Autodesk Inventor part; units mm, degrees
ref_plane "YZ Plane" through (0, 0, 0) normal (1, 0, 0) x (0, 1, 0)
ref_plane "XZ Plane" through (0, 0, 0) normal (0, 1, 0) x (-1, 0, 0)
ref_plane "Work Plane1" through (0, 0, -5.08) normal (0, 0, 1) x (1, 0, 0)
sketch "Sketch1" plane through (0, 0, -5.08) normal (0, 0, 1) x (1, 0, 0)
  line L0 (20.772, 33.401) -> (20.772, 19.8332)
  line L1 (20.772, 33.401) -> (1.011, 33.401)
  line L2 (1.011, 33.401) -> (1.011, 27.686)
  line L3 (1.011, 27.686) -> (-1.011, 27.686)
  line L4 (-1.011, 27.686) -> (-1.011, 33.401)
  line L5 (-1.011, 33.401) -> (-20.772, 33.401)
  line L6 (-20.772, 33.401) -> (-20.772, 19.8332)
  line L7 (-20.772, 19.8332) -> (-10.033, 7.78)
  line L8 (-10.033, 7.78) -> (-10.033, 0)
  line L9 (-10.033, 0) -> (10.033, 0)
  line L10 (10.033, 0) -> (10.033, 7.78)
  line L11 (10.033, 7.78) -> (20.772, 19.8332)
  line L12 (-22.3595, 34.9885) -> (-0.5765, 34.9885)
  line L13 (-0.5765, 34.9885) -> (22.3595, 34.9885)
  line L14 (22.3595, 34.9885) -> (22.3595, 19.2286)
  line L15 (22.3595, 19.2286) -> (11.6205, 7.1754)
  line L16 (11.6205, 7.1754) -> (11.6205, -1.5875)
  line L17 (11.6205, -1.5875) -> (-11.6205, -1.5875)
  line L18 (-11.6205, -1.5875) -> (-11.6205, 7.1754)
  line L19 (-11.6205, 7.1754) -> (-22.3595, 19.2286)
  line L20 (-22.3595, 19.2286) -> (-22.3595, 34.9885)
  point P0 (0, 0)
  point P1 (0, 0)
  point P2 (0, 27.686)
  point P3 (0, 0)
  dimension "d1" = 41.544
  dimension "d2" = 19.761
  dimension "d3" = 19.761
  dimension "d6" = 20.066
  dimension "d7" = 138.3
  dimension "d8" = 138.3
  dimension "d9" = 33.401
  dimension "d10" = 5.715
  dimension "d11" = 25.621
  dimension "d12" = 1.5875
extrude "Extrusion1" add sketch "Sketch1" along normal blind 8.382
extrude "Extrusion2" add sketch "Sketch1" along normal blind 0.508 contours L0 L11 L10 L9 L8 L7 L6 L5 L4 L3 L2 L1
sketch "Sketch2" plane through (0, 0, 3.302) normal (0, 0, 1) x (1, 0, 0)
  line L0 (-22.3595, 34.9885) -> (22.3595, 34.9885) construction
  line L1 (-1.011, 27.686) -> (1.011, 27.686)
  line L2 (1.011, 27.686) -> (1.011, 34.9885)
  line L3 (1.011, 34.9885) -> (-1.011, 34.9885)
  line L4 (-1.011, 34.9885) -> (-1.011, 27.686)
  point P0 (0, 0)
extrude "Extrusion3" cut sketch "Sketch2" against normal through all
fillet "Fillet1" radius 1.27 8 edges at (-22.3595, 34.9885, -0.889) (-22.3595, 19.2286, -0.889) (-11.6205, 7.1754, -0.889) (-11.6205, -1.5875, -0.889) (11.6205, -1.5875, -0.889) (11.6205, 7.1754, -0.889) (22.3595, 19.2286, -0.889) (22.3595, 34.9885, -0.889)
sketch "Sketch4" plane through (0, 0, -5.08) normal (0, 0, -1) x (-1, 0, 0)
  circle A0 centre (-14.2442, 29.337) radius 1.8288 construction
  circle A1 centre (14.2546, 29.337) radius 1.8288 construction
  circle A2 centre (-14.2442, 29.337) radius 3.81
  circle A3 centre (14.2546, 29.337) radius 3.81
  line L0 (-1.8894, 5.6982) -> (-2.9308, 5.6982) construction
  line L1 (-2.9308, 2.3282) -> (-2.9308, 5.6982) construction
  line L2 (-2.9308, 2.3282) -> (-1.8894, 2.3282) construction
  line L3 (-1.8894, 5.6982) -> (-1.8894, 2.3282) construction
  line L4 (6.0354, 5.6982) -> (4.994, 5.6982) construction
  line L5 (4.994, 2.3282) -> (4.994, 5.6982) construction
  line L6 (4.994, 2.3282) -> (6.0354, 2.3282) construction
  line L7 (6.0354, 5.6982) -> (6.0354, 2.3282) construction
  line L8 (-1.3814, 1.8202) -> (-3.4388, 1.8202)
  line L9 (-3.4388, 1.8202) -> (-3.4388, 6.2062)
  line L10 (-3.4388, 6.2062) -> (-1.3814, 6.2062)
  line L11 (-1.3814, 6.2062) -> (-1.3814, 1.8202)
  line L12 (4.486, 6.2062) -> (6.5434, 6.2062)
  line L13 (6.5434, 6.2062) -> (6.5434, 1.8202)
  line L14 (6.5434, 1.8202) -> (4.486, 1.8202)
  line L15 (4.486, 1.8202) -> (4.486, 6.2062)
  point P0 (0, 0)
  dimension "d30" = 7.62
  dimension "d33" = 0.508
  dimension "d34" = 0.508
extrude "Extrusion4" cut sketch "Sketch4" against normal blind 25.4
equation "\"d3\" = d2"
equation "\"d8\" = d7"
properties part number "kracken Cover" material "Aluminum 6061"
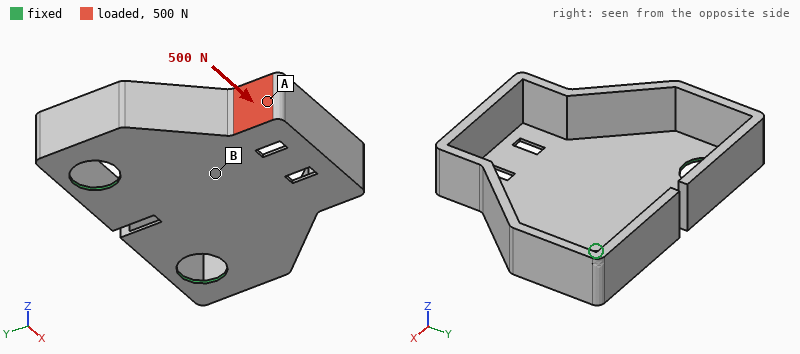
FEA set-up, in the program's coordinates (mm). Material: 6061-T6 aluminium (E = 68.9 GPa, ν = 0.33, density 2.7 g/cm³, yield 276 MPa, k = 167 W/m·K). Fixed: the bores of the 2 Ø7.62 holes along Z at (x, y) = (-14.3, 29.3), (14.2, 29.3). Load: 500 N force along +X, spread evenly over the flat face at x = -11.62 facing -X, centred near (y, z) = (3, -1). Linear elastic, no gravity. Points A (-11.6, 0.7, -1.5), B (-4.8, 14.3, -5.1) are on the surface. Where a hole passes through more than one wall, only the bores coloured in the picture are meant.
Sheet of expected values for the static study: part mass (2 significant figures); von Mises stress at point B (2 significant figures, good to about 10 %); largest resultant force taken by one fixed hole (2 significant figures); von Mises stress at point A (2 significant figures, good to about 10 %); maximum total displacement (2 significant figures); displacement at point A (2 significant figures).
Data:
6.4 g
56 MPa
440 N
120 MPa
0.39 mm
0.28 mm
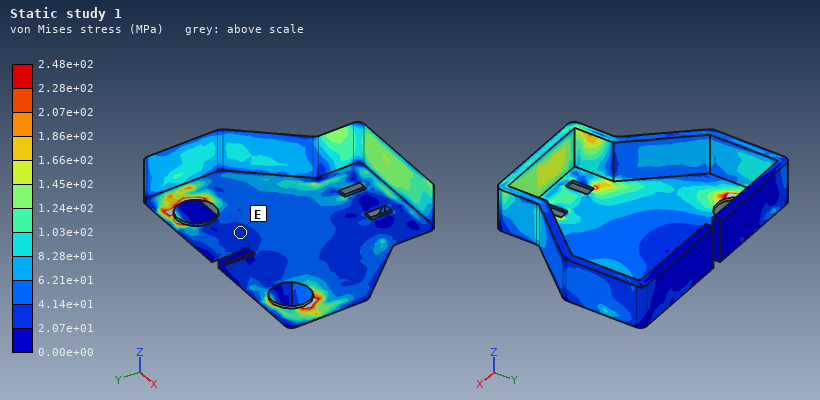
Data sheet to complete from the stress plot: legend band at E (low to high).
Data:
2.07e+01 to 4.14e+01 MPa
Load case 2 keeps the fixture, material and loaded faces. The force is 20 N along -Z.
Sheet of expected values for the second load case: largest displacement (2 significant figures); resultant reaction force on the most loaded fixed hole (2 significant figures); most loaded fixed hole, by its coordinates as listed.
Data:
0.21 mm
15 N
(-14.3, 29.3)
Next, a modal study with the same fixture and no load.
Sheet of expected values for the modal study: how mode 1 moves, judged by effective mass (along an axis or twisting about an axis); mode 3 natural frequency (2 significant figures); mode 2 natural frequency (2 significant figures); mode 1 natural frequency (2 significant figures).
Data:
along Z
4900 Hz
3100 Hz
1200 Hz
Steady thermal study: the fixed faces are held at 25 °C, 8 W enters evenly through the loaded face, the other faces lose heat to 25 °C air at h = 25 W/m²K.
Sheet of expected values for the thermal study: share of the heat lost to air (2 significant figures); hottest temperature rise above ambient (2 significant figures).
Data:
18 %
42 K
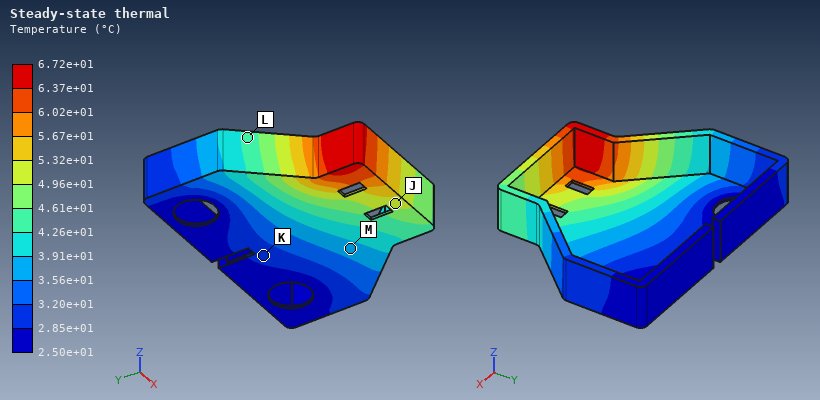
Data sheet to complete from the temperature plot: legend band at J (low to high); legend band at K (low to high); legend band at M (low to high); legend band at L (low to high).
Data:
4.96e+01 to 5.32e+01 °C
2.85e+01 to 3.20e+01 °C
3.56e+01 to 3.91e+01 °C
4.26e+01 to 4.61e+01 °C
